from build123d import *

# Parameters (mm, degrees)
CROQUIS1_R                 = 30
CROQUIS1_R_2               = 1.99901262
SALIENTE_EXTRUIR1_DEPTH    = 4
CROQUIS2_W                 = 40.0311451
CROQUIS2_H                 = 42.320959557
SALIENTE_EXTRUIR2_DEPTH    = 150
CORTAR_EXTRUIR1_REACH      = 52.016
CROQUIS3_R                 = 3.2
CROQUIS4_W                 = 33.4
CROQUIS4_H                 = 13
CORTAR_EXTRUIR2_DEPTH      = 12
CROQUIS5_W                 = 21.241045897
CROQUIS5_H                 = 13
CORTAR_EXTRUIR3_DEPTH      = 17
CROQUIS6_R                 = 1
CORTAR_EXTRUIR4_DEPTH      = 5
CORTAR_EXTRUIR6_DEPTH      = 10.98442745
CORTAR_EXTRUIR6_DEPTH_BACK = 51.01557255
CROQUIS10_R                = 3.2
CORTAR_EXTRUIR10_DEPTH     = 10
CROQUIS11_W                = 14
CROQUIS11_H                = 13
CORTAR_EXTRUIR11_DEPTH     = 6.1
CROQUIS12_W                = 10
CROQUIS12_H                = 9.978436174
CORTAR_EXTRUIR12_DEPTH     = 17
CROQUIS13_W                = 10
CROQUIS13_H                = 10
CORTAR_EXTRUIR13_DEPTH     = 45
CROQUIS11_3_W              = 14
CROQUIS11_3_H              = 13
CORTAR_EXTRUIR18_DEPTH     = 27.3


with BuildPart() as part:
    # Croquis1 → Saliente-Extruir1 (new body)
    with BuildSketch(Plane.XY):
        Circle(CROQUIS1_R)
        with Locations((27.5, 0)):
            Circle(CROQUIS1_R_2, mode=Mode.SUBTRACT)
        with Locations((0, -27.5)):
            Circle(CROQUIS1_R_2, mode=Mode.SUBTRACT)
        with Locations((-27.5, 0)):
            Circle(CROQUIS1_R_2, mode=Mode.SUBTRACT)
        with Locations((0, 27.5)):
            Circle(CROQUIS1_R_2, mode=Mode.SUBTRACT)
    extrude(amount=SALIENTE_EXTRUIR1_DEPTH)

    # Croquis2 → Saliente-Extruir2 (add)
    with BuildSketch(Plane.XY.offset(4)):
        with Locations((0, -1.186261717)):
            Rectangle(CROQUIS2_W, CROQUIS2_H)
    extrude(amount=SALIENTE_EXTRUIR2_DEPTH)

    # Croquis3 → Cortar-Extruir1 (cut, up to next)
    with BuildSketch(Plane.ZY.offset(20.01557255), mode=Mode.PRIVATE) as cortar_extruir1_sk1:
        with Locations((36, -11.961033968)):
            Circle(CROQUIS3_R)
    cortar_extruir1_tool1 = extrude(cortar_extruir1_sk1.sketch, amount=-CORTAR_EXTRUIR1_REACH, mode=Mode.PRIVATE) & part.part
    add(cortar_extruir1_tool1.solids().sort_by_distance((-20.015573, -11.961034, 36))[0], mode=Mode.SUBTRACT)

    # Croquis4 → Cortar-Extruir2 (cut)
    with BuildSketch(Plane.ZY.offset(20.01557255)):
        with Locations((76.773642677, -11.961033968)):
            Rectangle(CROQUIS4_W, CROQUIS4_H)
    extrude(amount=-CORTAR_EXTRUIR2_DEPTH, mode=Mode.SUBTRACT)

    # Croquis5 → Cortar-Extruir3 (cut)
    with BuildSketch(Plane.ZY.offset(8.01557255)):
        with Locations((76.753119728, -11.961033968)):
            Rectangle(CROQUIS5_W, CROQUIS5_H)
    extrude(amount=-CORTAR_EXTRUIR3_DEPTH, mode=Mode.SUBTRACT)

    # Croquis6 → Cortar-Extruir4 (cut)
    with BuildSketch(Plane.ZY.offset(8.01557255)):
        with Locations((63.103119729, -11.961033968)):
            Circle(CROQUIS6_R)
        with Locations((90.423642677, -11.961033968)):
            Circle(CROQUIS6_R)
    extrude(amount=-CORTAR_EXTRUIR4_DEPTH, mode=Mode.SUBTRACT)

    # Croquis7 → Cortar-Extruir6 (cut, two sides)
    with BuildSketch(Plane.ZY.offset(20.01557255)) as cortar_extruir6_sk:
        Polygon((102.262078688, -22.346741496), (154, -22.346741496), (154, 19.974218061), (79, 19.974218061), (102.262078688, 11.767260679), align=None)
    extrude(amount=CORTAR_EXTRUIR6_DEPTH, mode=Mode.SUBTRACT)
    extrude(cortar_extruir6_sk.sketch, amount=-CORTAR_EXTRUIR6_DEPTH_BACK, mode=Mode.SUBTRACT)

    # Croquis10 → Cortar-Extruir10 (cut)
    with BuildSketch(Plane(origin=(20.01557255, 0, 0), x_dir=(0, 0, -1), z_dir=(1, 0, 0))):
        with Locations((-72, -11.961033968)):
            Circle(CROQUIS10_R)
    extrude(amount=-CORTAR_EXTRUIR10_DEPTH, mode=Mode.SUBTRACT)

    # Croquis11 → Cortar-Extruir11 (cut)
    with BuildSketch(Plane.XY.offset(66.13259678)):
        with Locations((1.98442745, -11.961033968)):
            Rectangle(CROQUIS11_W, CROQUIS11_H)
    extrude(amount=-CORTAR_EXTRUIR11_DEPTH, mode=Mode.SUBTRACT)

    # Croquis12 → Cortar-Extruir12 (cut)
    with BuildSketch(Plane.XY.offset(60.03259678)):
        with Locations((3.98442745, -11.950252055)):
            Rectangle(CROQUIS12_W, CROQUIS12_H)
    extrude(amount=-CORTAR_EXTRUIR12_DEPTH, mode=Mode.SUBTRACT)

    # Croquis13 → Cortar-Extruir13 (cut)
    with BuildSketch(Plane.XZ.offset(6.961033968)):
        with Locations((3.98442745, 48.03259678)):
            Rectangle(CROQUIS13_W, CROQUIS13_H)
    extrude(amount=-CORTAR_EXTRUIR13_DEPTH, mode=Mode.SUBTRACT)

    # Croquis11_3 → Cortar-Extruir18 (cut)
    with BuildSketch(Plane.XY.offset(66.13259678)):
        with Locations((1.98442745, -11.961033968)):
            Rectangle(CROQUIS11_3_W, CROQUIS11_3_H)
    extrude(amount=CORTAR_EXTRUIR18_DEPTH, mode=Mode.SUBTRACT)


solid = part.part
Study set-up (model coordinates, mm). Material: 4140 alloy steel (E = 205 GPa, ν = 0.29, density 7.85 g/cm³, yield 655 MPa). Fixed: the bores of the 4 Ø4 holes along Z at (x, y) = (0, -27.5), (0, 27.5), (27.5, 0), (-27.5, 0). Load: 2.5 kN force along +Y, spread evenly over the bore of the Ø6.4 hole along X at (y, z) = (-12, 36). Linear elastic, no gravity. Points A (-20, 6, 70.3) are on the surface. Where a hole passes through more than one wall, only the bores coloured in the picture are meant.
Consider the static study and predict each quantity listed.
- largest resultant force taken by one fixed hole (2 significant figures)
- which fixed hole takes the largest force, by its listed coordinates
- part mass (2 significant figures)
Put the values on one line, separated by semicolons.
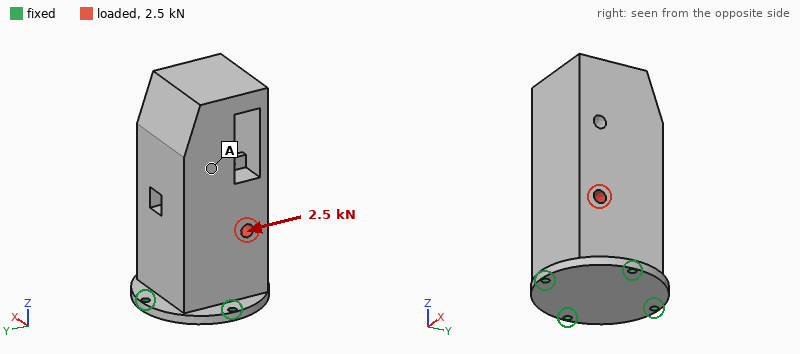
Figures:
2.2 kN; (0, -27.5); 1.2 kg
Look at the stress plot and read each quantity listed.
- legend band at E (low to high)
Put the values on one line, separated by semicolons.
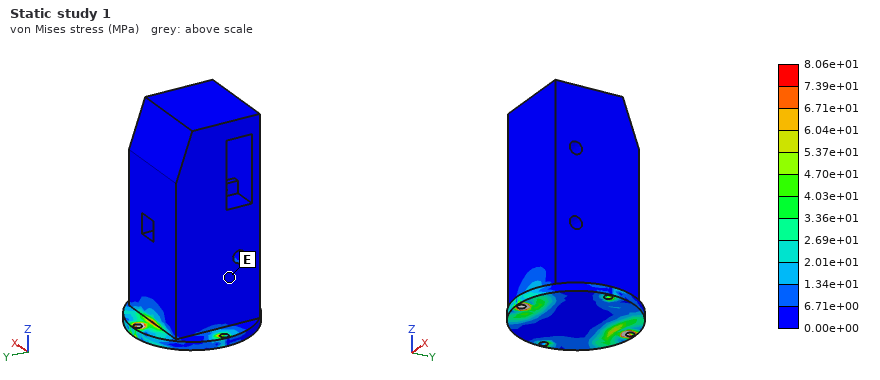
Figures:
0.00e+00 to 6.71e+00 MPa
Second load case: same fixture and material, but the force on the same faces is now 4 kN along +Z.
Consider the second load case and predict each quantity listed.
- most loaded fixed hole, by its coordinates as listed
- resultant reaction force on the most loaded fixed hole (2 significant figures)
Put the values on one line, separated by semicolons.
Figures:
(0, -27.5); 2.2 kN
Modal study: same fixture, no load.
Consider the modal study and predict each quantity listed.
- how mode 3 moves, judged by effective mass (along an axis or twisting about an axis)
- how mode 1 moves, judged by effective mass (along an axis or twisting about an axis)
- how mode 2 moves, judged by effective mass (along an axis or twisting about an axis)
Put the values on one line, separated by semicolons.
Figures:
along Z; along X; along Y
